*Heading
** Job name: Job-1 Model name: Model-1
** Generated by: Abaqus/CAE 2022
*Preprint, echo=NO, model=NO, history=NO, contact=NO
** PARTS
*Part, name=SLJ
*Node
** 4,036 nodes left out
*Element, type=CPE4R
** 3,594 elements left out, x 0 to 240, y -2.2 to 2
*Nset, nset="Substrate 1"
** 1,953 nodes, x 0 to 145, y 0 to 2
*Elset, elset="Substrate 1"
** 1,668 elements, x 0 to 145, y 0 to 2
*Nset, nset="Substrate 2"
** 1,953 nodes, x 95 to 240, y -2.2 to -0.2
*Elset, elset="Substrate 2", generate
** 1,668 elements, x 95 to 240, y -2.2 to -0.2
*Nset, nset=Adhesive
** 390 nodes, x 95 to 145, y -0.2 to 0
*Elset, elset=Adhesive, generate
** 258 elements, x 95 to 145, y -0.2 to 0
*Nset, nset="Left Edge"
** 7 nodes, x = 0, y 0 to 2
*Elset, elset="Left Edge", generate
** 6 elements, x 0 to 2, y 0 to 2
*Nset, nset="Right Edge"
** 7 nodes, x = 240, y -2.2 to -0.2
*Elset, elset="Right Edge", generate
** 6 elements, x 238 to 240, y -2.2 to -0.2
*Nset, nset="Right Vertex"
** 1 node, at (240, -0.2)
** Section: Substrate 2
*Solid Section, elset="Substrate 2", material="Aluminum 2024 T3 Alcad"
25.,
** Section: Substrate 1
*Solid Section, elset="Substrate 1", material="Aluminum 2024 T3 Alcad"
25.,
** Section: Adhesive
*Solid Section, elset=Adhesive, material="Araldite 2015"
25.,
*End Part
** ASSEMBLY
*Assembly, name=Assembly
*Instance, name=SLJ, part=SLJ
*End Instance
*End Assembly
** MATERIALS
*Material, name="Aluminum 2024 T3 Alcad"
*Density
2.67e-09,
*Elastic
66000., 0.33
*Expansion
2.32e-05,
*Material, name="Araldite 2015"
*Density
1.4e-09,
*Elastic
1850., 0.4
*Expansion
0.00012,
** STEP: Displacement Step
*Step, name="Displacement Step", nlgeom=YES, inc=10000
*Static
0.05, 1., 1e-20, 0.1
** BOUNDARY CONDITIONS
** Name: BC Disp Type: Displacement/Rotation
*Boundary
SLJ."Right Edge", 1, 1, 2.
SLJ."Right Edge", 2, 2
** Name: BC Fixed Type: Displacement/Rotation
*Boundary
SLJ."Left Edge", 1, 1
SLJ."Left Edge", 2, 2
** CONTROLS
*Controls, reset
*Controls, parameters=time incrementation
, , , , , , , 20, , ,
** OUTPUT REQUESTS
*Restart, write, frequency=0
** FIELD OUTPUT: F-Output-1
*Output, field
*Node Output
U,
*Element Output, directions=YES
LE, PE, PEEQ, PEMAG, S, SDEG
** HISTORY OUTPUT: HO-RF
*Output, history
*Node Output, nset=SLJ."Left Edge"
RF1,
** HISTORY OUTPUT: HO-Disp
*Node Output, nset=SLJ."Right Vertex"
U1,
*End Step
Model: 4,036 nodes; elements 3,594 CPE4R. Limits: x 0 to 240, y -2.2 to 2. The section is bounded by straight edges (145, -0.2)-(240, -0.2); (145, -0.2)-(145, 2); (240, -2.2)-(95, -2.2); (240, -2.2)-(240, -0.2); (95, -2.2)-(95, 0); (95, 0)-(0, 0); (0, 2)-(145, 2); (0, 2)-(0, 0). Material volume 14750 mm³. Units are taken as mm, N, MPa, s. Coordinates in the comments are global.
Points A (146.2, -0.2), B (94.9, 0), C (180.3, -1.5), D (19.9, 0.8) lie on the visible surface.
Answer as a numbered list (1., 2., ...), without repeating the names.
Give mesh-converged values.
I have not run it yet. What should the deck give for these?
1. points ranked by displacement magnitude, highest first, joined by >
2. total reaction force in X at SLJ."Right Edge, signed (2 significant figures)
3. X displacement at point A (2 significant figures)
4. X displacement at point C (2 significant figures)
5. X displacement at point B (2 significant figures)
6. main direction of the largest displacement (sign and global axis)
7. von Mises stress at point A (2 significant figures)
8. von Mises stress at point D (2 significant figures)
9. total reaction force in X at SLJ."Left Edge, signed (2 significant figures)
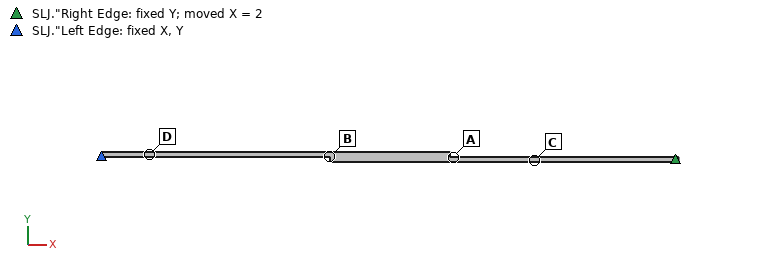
1. C > A > B > D
2. 33000 N
3. 1.1 mm
4. 1.5 mm
5. 0.87 mm
6. +X
7. 920 MPa
8. 590 MPa
9. -33000 N
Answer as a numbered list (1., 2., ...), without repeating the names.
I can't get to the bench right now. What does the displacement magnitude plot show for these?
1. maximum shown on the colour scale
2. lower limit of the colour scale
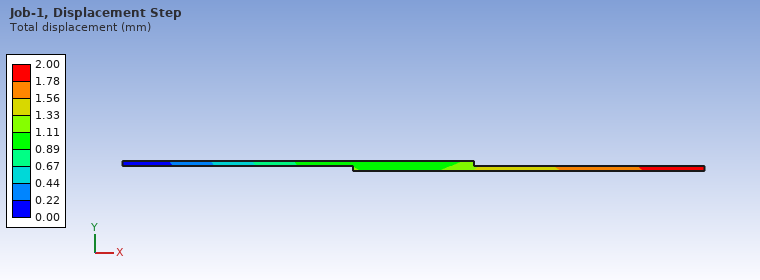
1. 2.00 mm
2. 0.00 mm
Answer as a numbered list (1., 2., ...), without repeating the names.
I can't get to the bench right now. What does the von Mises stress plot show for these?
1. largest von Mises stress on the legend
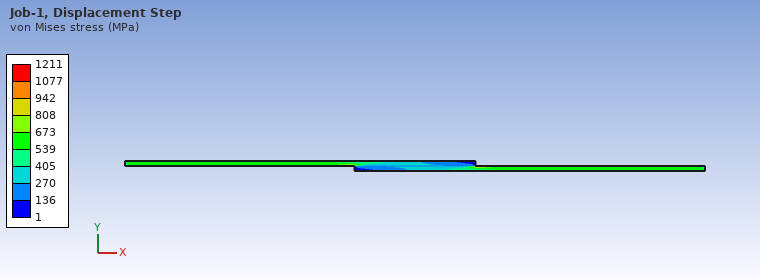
1. 1211 MPa
